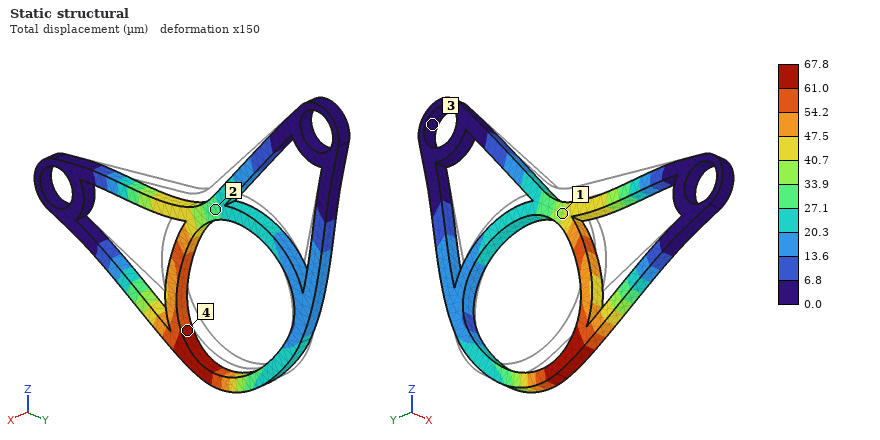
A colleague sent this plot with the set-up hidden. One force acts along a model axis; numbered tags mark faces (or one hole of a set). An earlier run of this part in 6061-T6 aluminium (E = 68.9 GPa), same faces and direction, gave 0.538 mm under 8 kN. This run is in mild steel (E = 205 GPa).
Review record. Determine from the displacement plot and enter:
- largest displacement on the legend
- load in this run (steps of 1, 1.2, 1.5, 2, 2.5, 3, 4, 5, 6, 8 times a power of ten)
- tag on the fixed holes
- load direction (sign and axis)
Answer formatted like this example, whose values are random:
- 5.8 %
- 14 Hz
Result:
- 67.8 µm
- 3 kN
- 3
- -Z
